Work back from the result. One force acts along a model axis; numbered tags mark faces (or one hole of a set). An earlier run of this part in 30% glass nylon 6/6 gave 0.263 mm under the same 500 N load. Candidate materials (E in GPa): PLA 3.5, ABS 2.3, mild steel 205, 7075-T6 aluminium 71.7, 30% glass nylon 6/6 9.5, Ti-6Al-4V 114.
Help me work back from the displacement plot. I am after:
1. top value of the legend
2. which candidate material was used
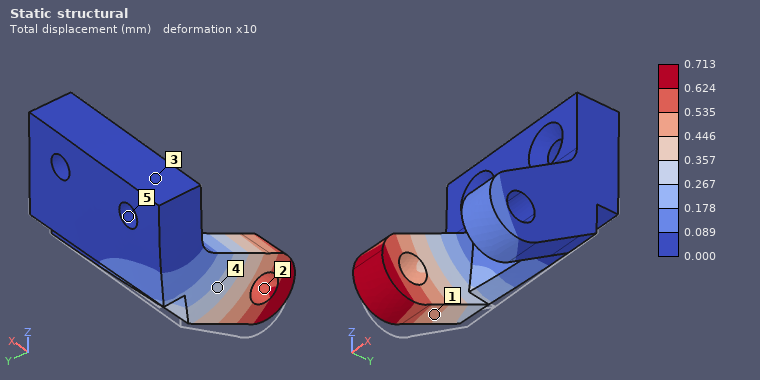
0.713 mm
PLA
